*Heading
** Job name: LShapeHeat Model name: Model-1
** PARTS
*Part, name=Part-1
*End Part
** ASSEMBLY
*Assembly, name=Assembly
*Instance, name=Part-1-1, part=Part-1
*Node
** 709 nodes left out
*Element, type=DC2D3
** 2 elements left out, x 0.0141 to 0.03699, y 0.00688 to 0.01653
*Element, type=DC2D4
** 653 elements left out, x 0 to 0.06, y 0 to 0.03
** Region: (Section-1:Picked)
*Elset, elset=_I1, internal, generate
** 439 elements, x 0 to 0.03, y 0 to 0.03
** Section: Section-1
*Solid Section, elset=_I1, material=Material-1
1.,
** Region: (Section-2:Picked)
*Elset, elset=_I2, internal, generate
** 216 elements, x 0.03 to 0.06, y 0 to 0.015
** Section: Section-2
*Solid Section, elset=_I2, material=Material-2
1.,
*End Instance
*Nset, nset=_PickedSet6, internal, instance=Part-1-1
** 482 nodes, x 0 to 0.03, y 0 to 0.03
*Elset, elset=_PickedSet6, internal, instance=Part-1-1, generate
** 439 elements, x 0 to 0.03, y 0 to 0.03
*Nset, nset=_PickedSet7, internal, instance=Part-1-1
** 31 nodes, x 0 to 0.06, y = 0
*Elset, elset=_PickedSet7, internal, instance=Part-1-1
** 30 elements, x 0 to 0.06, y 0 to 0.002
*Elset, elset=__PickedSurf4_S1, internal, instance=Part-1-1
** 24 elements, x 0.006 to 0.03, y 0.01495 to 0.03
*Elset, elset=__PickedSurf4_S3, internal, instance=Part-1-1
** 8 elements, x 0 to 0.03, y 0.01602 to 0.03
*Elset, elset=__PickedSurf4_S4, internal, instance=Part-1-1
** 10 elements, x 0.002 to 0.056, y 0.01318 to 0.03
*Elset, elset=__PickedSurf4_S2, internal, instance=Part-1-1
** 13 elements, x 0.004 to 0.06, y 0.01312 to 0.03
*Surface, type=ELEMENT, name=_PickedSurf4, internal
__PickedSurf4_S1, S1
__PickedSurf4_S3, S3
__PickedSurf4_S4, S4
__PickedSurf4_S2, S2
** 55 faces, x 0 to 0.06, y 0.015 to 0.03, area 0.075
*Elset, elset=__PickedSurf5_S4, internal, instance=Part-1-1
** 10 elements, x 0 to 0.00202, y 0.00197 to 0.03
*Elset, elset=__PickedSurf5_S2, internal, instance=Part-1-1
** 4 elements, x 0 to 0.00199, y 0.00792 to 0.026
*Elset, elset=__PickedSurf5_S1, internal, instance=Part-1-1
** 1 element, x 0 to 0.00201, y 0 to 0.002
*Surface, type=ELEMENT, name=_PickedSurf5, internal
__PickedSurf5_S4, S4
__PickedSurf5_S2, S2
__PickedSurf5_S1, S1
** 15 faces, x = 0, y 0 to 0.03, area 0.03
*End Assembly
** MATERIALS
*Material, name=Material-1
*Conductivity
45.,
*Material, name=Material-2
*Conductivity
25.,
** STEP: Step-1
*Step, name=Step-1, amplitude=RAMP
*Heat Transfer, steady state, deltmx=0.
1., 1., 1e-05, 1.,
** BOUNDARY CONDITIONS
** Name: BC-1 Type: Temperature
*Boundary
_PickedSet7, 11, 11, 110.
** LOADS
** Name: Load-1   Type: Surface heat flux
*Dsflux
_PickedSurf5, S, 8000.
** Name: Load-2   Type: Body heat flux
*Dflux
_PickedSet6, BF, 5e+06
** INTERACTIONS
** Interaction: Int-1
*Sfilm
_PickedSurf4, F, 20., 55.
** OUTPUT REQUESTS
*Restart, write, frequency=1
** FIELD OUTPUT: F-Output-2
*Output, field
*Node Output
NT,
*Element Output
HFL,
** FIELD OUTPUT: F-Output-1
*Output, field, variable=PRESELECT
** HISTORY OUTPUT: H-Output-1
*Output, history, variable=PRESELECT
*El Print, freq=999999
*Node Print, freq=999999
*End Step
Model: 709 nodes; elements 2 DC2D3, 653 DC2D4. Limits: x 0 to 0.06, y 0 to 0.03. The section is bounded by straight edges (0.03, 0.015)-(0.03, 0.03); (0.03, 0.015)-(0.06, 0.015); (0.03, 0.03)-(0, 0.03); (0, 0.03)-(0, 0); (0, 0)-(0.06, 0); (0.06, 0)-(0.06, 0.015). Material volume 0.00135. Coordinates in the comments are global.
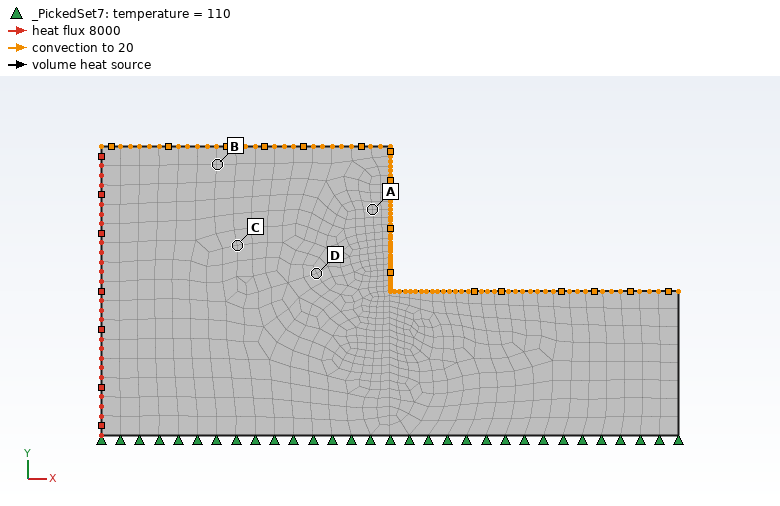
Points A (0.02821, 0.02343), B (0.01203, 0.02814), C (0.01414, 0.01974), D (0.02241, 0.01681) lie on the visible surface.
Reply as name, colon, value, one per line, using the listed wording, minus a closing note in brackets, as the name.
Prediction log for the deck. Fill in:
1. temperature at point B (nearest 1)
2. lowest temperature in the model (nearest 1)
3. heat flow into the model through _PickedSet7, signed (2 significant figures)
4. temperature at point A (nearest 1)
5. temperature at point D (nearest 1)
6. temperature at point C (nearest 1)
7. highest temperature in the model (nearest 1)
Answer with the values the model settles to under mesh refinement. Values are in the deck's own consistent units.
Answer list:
temperature at point B: 153
lowest temperature in the model: 109
heat flow into the model through _PickedSet7, signed: -4200
temperature at point A: 147
temperature at point D: 142
temperature at point C: 148
highest temperature in the model: 155
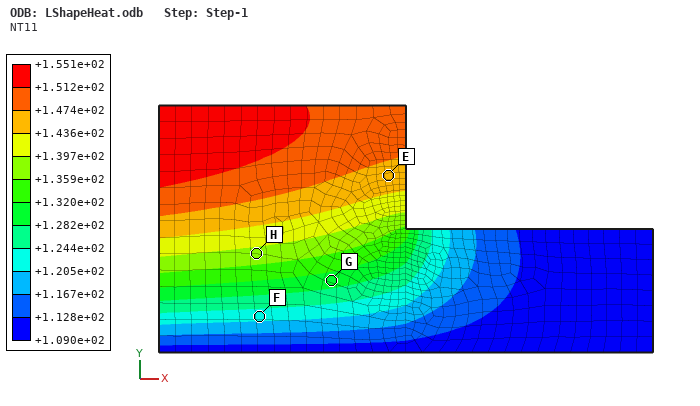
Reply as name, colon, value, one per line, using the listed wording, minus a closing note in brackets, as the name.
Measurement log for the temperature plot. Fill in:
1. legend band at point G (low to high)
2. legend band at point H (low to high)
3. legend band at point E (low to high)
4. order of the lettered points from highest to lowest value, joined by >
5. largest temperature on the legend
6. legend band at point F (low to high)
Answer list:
legend band at point G: +1.282e+02 to +1.320e+02
legend band at point H: +1.359e+02 to +1.397e+02
legend band at point E: +1.436e+02 to +1.474e+02
order of the lettered points from highest to lowest value, joined by >: E > H > G > F
largest temperature on the legend: +1.551e+02
legend band at point F: +1.205e+02 to +1.244e+02
